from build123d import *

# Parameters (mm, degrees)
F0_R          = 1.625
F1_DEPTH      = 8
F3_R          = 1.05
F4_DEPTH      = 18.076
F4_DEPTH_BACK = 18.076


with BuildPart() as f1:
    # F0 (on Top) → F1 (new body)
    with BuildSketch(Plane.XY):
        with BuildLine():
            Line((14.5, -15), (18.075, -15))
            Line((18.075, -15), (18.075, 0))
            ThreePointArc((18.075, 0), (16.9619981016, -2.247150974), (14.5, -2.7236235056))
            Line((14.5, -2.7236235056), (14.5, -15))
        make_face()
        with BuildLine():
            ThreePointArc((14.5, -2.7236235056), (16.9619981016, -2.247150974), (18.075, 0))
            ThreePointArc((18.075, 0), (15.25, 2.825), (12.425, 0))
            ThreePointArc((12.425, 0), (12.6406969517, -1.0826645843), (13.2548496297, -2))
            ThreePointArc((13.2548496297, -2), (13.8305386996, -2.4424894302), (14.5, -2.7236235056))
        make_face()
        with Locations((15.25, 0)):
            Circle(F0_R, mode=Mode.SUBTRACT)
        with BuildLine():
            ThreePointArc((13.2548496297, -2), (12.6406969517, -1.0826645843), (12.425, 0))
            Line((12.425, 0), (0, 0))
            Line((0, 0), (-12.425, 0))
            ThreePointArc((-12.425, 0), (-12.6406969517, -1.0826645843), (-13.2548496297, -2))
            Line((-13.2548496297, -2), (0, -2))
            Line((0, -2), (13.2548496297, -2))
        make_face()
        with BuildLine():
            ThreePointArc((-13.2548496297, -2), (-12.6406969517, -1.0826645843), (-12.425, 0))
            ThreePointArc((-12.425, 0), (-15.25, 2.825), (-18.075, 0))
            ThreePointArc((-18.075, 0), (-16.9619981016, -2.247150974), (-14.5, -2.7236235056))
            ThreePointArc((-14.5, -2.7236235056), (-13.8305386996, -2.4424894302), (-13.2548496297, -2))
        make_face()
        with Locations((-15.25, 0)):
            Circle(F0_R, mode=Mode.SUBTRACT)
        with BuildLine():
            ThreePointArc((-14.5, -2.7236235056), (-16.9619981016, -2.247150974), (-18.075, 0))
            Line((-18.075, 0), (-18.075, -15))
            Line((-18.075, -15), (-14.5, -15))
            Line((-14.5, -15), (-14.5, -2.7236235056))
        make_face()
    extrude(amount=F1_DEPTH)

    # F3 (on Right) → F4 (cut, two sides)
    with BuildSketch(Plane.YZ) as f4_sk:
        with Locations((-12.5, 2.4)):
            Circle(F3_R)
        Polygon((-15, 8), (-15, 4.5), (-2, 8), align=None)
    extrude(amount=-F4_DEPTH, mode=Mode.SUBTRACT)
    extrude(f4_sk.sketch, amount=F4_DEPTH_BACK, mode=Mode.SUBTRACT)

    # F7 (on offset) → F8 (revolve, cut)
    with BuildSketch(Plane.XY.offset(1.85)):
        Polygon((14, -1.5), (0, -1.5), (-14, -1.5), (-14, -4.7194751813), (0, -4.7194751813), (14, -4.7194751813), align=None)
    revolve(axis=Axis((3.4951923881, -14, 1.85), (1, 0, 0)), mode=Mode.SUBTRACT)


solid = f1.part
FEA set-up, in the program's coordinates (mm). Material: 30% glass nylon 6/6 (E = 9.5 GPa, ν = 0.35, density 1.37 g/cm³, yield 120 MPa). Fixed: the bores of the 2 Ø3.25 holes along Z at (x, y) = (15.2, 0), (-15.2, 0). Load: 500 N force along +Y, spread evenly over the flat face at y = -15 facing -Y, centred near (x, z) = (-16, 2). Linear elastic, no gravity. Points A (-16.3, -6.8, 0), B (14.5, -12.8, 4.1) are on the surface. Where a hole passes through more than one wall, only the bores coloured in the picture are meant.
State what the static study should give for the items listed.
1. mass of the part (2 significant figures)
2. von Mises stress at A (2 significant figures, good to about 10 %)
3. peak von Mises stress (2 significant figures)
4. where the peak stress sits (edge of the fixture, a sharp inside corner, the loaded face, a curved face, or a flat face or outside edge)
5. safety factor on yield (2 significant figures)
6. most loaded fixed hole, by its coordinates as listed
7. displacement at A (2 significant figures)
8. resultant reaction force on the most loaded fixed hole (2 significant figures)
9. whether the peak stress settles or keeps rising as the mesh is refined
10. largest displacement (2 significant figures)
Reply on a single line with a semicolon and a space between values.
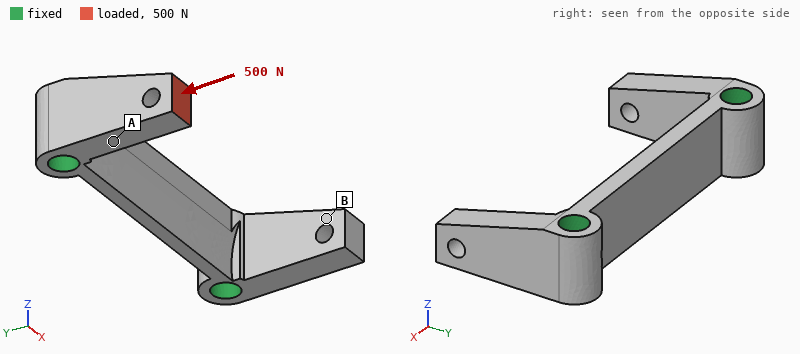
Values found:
1.6 g; 42 MPa; 130 MPa; a curved face; 0.93; (-15.2, 0); 30 µm; 500 N; settles; 92 µm
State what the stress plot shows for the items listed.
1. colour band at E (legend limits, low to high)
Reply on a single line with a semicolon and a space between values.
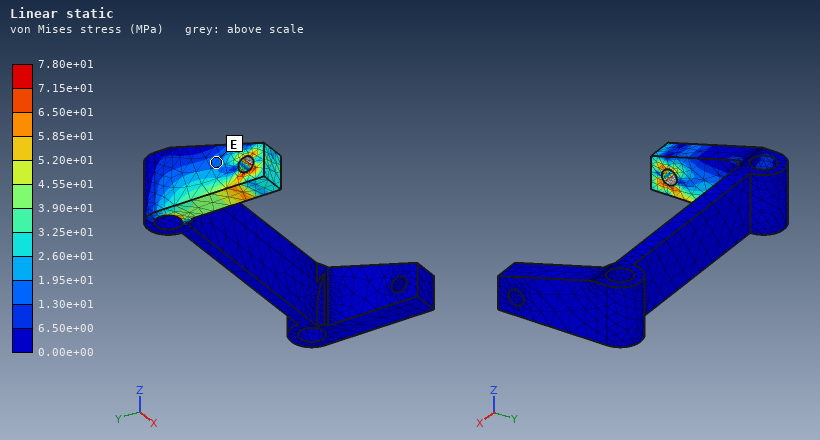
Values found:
1.30e+01 to 1.95e+01 MPa
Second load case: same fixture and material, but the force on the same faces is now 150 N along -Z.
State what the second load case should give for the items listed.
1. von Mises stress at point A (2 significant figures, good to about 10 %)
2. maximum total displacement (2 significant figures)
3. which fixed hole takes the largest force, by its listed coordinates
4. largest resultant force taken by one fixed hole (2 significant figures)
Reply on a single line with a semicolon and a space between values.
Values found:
46 MPa; 0.19 mm; (-15.2, 0); 150 N
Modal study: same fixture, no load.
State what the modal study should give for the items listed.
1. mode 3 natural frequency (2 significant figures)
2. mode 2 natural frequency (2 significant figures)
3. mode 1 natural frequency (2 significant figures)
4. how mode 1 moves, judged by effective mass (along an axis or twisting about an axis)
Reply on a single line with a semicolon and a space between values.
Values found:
9500 Hz; 9500 Hz; 6800 Hz; along Y
